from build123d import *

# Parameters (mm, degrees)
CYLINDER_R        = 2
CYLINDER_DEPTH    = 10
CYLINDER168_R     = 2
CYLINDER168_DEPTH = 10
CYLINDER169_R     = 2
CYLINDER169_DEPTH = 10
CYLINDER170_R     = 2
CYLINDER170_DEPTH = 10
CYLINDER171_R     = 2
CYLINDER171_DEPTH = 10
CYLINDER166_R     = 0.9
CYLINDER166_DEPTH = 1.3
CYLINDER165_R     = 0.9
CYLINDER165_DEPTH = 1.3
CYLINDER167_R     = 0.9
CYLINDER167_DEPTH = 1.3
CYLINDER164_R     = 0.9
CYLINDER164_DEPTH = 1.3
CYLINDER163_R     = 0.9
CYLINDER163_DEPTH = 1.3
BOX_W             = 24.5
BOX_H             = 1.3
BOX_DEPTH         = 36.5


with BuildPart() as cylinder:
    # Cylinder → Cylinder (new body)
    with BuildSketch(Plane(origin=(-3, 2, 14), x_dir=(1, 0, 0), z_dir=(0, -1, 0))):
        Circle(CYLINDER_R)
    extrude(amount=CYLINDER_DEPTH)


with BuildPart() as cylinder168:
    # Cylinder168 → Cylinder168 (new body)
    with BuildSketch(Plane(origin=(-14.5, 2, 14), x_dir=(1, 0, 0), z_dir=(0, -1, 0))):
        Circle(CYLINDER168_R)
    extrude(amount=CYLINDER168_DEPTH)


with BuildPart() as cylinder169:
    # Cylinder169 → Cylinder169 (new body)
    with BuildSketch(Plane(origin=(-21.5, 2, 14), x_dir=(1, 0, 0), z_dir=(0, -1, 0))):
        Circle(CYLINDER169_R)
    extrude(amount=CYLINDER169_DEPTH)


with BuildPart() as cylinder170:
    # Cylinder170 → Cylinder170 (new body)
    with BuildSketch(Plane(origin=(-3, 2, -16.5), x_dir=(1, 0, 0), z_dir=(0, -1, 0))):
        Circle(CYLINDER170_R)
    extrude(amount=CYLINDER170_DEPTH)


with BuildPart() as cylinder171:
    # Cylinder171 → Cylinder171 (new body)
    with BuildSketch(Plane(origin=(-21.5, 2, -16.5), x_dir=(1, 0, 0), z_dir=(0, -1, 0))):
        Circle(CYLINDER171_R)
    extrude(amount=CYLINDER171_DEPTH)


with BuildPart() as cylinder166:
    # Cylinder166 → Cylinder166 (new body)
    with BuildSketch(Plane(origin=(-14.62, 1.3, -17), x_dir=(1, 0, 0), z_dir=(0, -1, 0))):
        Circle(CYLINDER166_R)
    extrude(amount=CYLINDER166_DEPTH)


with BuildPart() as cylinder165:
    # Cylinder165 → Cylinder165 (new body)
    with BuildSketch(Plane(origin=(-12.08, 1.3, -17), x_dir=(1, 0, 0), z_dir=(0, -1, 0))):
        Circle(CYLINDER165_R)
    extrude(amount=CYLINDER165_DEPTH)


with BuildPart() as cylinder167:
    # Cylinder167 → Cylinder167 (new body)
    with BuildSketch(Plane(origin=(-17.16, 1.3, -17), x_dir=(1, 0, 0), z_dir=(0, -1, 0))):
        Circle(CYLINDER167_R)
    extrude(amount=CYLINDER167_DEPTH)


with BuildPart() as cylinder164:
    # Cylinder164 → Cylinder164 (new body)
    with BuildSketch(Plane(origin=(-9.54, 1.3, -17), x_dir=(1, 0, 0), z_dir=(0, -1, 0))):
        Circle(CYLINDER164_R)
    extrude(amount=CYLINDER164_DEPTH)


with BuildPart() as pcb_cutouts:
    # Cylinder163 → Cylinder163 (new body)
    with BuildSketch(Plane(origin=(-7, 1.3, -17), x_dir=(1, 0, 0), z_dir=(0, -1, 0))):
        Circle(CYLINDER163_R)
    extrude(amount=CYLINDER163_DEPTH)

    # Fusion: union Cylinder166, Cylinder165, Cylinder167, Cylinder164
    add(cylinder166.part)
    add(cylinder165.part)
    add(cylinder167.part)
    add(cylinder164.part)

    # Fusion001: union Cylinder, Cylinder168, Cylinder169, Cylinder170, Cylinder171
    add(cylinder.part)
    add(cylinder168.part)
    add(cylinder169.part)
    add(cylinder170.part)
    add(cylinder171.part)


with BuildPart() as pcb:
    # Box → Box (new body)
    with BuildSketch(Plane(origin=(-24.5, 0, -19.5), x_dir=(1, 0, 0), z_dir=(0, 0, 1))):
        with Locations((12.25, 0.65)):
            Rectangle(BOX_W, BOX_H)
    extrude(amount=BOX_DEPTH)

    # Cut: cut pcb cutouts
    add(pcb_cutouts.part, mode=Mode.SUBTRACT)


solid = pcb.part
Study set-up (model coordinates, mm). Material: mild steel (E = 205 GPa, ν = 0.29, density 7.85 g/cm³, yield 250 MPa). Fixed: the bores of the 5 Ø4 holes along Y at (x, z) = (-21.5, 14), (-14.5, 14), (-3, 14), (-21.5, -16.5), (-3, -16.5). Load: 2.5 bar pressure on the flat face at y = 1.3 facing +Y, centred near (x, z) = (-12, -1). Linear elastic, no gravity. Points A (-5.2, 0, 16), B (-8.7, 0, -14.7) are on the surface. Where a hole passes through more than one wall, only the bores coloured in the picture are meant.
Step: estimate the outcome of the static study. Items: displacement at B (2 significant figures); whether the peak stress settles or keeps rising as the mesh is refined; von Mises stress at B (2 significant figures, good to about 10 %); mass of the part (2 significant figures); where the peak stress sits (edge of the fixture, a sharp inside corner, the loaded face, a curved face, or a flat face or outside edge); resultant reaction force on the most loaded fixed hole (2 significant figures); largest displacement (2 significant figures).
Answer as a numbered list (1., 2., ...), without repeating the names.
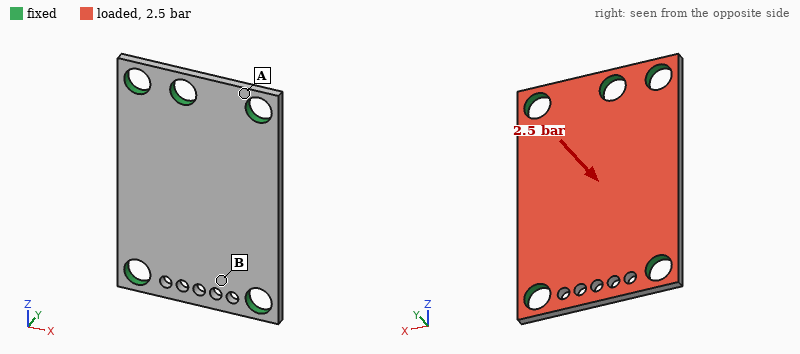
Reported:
1. 1.9 µm
2. keeps rising
3. 18 MPa
4. 8.4 g
5. edge of the fixture
6. 50 N
7. 12 µm
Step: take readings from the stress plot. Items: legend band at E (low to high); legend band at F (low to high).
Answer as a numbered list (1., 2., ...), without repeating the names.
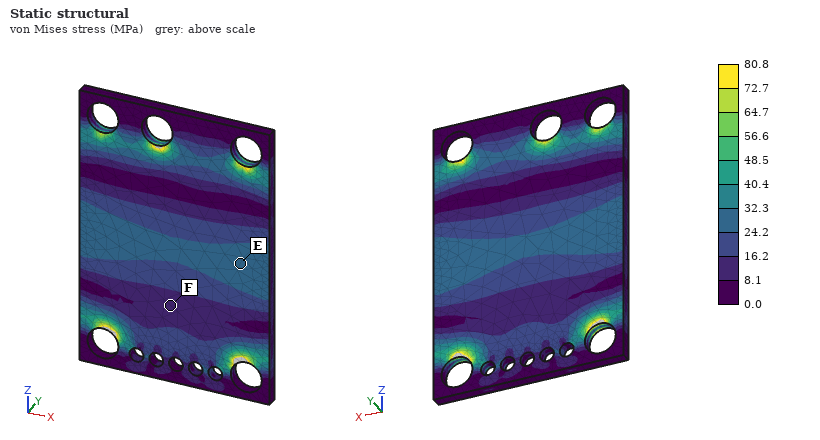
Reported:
1. 24.2 to 32.3 MPa
2. 8.1 to 16.2 MPa
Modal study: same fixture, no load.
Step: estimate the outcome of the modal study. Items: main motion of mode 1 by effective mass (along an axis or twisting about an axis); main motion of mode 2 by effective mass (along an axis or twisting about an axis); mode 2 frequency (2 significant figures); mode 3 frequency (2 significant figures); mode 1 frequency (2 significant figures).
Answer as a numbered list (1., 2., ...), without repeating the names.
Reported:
1. along Y
2. twisting about Z
3. 11 kHz
4. 18 kHz
5. 8500 Hz
